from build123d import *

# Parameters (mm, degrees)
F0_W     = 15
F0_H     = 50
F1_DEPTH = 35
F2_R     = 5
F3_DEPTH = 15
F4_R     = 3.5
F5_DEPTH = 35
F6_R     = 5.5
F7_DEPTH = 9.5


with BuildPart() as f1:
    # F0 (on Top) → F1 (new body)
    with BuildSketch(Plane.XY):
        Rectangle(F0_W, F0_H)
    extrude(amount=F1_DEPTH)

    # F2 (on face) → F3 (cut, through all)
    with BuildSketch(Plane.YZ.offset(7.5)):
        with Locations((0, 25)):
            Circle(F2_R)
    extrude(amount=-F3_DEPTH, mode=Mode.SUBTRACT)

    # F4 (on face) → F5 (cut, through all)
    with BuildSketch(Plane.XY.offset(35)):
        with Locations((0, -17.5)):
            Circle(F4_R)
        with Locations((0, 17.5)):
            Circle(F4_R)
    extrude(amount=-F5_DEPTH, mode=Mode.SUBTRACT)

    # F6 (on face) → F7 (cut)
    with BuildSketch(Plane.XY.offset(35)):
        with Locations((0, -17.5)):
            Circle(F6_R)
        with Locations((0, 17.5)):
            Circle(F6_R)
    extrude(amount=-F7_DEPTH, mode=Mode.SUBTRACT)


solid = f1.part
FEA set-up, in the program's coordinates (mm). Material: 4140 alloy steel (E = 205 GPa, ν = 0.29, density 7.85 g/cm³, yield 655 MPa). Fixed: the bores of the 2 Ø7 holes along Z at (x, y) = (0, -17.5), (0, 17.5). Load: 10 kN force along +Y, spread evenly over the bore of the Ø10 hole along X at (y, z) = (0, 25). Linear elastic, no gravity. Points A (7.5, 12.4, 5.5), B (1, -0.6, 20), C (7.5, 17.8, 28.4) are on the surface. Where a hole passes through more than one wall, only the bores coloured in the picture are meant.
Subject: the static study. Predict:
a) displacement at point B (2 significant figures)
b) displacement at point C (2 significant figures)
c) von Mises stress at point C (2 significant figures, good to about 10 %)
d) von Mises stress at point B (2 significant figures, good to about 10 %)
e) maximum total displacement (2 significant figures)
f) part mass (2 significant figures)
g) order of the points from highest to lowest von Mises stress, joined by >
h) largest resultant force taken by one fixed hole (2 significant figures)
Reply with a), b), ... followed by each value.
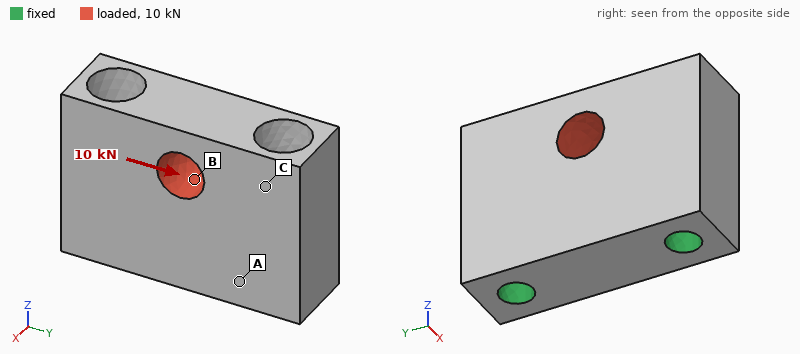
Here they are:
a) 1.2 µm
b) 1.4 µm
c) 16 MPa
d) 37 MPa
e) 3.3 µm
f) 170 g
g) B > C > A
h) 5.2 kN
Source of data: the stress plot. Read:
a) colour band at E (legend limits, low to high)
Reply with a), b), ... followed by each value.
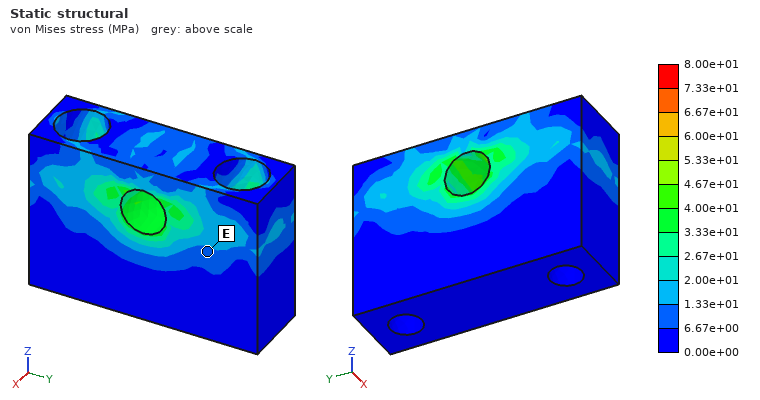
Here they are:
a) 6.67e+00 to 1.33e+01 MPa
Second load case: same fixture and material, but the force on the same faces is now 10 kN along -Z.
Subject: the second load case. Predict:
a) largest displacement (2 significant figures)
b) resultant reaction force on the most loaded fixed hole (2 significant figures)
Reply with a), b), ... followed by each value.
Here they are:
a) 4.1 µm
b) 5.3 kN
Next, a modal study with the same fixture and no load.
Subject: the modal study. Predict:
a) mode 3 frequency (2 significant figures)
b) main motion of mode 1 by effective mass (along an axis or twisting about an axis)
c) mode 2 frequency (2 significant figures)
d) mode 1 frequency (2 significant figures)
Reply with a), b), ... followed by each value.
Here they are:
a) 39 kHz
b) along X
c) 38 kHz
d) 25 kHz
